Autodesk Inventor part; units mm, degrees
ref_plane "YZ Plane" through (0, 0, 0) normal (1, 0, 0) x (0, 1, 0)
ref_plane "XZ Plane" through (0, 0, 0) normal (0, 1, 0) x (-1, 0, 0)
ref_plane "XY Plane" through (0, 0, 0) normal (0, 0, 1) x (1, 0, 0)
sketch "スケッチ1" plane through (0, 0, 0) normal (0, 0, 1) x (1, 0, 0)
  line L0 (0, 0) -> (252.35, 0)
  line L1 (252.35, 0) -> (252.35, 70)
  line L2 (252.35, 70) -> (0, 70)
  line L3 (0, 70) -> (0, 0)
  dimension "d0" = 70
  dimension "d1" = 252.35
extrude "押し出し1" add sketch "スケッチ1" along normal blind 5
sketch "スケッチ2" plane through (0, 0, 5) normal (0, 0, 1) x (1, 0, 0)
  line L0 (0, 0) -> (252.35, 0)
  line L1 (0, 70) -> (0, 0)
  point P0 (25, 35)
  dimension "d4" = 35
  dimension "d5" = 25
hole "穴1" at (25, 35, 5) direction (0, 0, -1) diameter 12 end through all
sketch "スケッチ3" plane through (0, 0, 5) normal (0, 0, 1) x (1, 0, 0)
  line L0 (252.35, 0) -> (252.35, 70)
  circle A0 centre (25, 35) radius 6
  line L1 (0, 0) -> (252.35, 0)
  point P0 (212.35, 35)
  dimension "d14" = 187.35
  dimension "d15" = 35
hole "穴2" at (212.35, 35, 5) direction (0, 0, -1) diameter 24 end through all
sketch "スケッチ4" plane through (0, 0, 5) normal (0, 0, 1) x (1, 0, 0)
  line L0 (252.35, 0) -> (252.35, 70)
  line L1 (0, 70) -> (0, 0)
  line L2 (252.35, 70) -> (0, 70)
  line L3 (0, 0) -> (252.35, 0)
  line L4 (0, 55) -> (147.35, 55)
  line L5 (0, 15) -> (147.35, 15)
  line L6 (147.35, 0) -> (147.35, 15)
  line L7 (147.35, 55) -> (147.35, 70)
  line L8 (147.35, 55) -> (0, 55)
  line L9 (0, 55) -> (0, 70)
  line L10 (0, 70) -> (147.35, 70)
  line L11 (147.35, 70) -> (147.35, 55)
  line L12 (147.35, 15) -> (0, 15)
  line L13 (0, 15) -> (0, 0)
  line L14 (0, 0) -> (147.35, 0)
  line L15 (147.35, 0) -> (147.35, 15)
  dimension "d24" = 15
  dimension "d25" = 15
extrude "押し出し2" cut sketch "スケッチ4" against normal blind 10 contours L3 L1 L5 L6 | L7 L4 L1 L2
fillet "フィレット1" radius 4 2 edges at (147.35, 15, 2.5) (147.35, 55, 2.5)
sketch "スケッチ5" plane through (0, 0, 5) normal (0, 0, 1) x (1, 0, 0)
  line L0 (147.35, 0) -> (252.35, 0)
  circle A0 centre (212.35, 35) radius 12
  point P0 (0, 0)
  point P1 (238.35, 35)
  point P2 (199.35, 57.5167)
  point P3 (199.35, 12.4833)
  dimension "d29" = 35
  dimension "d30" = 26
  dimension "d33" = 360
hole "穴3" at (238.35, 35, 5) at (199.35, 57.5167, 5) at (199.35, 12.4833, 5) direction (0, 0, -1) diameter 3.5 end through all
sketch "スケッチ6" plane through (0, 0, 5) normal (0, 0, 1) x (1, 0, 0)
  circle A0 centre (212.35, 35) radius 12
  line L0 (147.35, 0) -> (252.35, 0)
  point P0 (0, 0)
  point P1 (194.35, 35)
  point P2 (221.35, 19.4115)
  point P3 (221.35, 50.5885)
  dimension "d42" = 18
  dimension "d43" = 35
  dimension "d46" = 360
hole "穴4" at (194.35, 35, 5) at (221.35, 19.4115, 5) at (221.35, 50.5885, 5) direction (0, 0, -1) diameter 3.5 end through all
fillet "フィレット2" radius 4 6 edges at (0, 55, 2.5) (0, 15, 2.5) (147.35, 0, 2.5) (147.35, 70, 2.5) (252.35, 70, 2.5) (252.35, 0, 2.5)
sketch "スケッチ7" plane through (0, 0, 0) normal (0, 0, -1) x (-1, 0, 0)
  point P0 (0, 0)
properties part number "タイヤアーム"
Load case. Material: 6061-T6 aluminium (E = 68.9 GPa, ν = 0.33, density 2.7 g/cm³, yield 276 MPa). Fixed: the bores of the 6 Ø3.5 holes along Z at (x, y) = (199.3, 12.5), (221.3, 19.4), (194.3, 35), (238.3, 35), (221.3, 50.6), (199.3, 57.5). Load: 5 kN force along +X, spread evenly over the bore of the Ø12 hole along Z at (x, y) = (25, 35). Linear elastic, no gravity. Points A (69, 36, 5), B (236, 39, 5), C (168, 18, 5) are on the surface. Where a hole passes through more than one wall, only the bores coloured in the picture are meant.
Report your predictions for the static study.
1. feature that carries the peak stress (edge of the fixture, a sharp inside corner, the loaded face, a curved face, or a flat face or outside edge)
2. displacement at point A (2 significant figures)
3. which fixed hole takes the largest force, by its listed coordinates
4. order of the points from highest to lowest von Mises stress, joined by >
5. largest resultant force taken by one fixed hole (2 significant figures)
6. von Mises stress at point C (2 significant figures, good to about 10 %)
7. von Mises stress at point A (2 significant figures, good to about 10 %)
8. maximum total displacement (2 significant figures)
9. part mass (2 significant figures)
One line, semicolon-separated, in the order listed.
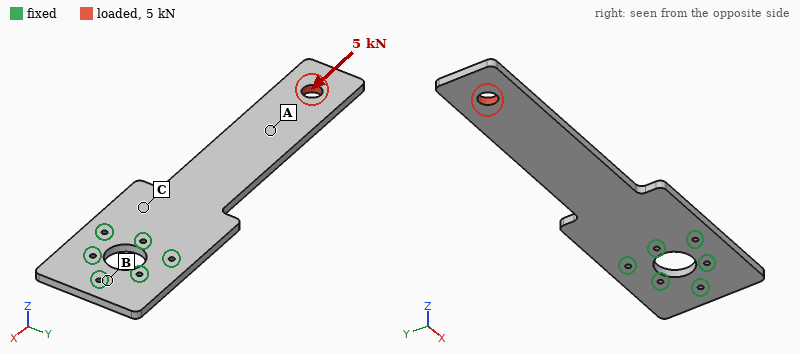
the loaded face; 42 µm; (194.3, 35); A > C > B; 1.6 kN; 17 MPa; 25 MPa; 65 µm; 170 g
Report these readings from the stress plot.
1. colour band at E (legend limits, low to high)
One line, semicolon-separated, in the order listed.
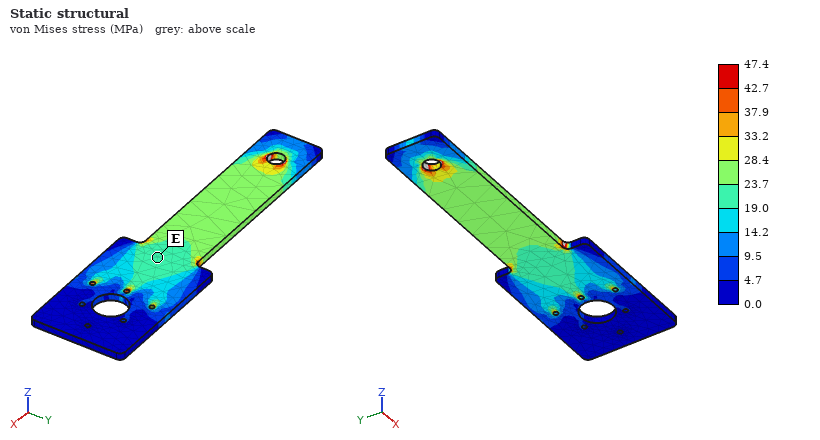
19.0 to 23.7 MPa
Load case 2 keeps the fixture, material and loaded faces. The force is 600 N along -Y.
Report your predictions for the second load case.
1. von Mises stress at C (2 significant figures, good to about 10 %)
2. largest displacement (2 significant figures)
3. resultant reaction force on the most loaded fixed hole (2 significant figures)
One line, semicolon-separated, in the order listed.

18 MPa; 0.42 mm; 1.7 kN
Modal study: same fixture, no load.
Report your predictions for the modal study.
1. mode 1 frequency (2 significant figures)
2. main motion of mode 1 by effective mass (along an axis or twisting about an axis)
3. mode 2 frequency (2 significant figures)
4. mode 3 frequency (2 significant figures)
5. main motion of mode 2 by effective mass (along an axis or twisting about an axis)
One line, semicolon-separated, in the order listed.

130 Hz; along Z; 710 Hz; 1100 Hz; along Z
